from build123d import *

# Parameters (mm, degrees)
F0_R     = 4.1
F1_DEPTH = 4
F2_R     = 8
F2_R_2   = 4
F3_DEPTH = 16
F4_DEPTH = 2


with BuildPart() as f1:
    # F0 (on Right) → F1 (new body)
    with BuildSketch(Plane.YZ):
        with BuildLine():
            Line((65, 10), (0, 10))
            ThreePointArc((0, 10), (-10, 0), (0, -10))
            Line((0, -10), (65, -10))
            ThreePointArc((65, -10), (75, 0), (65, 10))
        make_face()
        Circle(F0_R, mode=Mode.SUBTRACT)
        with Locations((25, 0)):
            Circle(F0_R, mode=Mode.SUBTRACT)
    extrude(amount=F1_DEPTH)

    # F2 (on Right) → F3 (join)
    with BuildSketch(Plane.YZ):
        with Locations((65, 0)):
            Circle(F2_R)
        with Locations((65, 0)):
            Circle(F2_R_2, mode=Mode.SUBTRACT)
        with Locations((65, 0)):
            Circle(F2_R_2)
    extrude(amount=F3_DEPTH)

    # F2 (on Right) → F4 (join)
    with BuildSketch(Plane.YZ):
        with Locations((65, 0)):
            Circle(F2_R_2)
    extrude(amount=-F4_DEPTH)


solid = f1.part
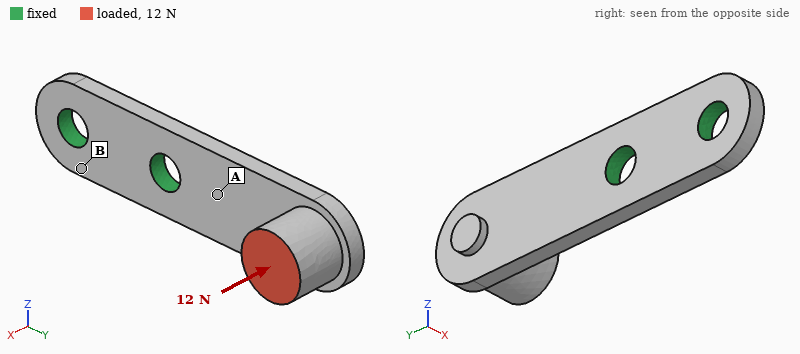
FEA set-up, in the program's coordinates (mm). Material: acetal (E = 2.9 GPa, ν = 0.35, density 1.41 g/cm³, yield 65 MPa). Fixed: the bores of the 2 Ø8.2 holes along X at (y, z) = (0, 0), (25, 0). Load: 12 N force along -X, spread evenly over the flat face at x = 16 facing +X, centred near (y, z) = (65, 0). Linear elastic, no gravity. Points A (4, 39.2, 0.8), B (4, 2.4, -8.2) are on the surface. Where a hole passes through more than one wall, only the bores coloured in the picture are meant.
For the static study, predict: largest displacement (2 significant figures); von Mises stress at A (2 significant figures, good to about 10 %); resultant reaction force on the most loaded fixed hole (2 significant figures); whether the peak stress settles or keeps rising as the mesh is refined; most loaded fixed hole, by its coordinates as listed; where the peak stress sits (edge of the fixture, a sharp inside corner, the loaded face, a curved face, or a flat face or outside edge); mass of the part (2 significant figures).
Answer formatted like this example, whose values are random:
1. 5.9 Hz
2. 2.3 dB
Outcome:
1. 0.92 mm
2. 5.3 MPa
3. 12 N
4. keeps rising
5. (25, 0)
6. edge of the fixture
7. 12 g
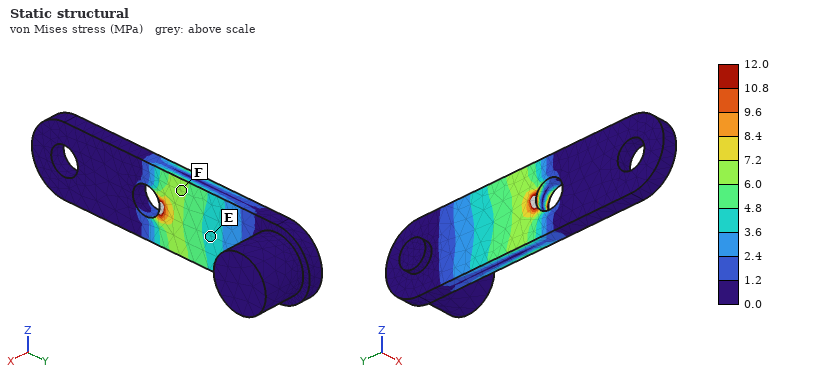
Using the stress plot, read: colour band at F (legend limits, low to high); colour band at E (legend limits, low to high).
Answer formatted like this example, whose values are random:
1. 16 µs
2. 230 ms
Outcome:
1. 6.0 to 7.2 MPa
2. 3.6 to 4.8 MPa
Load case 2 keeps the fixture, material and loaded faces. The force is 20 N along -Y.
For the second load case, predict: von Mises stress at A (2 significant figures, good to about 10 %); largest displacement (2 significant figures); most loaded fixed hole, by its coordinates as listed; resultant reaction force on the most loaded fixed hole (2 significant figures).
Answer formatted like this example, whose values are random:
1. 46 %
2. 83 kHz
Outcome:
1. 5.2 MPa
2. 0.91 mm
3. (25, 0)
4. 19 N
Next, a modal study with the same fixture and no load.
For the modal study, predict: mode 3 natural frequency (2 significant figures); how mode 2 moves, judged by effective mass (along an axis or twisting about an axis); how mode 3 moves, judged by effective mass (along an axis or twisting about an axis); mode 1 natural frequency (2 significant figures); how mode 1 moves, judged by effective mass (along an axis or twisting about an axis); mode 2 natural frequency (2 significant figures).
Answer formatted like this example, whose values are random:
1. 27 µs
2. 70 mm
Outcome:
1. 1500 Hz
2. along Z
3. along Z
4. 270 Hz
5. along X
6. 800 Hz
